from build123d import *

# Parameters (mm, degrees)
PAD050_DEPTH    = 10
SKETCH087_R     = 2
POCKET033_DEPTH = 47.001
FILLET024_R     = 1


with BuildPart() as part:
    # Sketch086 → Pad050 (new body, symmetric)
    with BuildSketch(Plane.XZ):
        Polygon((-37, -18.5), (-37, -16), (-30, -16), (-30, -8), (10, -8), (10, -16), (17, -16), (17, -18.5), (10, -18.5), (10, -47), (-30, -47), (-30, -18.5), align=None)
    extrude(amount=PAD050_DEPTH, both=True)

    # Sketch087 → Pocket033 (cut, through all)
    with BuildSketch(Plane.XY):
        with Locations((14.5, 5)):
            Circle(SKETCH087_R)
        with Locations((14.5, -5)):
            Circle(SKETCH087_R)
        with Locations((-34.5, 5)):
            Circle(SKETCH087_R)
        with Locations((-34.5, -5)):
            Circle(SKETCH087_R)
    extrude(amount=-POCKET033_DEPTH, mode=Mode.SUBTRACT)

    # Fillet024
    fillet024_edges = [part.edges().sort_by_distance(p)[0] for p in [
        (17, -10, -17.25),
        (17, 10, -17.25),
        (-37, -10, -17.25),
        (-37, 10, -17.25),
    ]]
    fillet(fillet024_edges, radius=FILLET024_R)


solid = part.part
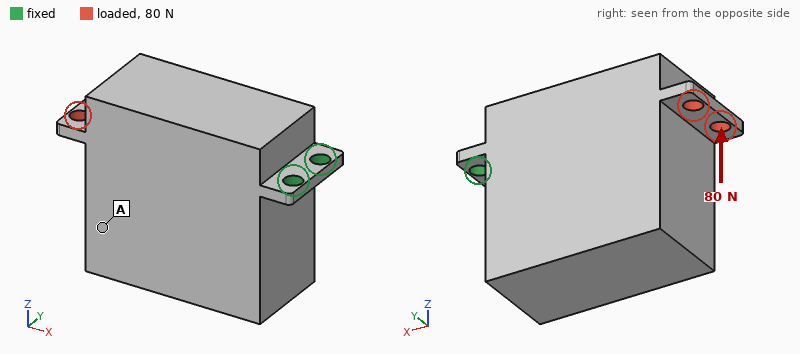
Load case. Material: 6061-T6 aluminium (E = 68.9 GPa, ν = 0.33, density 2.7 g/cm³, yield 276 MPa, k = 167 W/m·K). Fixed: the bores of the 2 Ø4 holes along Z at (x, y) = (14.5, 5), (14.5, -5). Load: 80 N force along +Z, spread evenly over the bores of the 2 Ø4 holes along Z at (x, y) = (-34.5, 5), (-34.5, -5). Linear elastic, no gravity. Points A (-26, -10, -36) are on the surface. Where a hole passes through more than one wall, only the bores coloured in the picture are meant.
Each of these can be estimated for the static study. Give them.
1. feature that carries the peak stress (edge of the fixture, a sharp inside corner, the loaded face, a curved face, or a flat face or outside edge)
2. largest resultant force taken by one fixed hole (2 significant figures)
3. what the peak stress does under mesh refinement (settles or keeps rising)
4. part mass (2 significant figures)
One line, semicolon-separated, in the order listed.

edge of the fixture; 40 N; keeps rising; 86 g
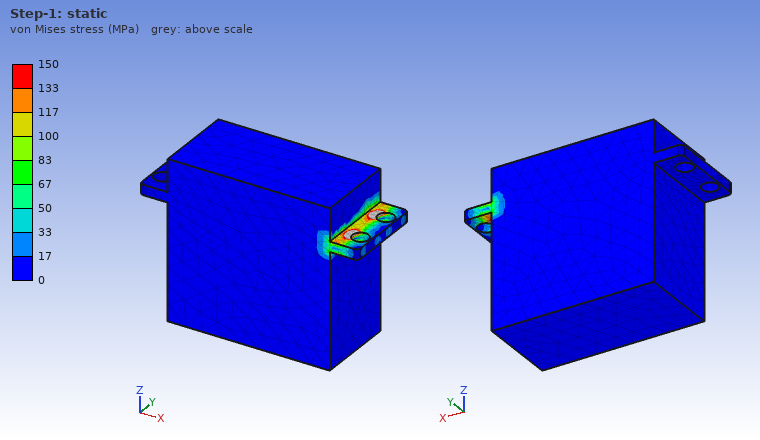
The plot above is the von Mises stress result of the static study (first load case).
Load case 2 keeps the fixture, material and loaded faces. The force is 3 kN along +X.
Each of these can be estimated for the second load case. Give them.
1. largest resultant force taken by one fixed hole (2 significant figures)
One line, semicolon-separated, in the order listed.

1.5 kN
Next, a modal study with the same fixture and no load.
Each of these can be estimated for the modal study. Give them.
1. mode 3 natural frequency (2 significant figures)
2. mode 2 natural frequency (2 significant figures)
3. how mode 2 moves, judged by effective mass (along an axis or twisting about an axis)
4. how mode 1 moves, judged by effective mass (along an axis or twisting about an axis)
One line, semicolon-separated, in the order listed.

3400 Hz; 1800 Hz; along Y; along Z
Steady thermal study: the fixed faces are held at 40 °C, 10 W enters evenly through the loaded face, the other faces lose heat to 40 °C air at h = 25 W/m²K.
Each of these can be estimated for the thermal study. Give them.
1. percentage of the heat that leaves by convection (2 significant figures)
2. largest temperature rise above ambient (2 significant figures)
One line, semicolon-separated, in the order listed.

13 %; 21 K
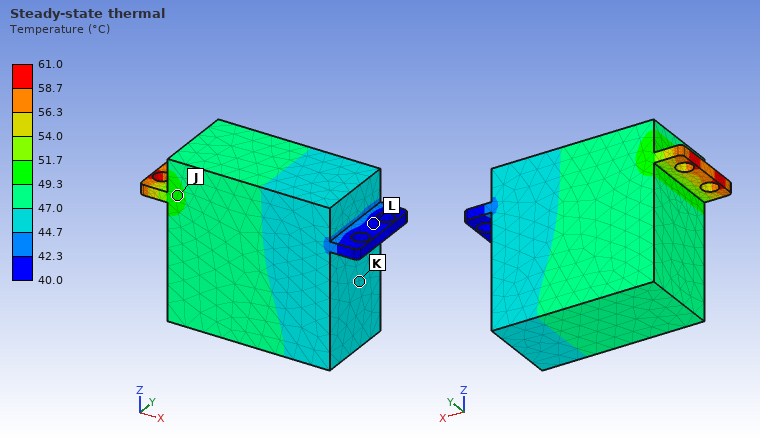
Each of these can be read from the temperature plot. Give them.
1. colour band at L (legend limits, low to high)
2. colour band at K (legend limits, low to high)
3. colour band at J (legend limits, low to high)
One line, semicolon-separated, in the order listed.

40.0 to 42.3 °C; 44.7 to 47.0 °C; 49.3 to 51.7 °C
